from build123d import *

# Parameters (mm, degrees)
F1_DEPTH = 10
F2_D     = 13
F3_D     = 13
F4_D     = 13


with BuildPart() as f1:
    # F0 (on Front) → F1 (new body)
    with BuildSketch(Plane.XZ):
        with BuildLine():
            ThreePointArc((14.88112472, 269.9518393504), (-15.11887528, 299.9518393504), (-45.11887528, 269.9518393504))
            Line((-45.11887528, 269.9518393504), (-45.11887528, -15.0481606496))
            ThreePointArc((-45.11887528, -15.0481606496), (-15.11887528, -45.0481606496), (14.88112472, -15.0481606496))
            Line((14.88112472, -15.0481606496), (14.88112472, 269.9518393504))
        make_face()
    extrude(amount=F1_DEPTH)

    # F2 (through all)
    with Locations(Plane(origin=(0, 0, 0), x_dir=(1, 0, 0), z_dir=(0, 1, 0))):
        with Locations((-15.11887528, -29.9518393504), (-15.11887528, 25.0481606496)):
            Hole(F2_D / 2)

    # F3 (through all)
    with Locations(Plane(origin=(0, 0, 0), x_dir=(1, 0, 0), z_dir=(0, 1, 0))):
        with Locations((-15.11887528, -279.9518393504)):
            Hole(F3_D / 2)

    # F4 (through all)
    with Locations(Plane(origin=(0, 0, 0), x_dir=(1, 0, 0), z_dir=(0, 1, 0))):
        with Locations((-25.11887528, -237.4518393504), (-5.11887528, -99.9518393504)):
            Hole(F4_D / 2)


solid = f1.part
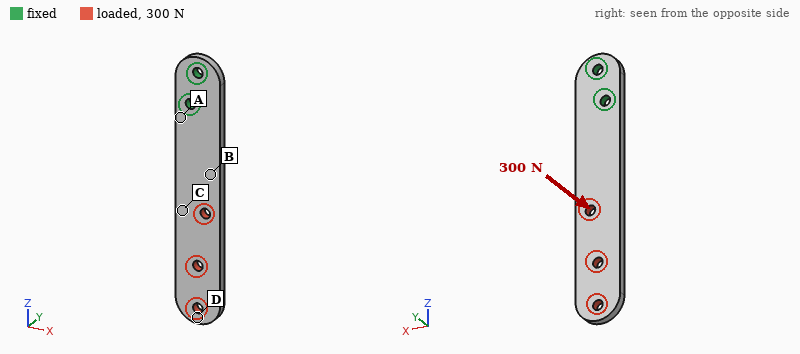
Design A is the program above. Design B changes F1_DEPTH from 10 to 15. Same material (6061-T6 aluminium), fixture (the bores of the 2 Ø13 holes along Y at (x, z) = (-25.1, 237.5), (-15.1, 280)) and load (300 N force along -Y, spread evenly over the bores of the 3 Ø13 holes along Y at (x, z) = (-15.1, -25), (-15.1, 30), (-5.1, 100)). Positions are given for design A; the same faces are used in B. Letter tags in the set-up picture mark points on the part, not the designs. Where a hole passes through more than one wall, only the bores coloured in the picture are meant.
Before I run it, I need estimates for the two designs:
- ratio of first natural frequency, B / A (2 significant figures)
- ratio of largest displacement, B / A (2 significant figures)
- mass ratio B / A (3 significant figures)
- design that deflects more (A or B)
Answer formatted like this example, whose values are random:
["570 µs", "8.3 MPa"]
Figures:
["1.5", "0.30", "1.50", "A"]
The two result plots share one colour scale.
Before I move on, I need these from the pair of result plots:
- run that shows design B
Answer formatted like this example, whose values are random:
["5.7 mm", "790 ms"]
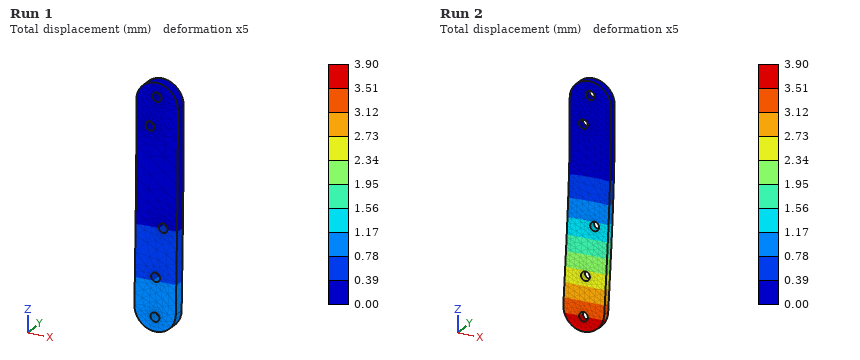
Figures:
["Run 1"]
